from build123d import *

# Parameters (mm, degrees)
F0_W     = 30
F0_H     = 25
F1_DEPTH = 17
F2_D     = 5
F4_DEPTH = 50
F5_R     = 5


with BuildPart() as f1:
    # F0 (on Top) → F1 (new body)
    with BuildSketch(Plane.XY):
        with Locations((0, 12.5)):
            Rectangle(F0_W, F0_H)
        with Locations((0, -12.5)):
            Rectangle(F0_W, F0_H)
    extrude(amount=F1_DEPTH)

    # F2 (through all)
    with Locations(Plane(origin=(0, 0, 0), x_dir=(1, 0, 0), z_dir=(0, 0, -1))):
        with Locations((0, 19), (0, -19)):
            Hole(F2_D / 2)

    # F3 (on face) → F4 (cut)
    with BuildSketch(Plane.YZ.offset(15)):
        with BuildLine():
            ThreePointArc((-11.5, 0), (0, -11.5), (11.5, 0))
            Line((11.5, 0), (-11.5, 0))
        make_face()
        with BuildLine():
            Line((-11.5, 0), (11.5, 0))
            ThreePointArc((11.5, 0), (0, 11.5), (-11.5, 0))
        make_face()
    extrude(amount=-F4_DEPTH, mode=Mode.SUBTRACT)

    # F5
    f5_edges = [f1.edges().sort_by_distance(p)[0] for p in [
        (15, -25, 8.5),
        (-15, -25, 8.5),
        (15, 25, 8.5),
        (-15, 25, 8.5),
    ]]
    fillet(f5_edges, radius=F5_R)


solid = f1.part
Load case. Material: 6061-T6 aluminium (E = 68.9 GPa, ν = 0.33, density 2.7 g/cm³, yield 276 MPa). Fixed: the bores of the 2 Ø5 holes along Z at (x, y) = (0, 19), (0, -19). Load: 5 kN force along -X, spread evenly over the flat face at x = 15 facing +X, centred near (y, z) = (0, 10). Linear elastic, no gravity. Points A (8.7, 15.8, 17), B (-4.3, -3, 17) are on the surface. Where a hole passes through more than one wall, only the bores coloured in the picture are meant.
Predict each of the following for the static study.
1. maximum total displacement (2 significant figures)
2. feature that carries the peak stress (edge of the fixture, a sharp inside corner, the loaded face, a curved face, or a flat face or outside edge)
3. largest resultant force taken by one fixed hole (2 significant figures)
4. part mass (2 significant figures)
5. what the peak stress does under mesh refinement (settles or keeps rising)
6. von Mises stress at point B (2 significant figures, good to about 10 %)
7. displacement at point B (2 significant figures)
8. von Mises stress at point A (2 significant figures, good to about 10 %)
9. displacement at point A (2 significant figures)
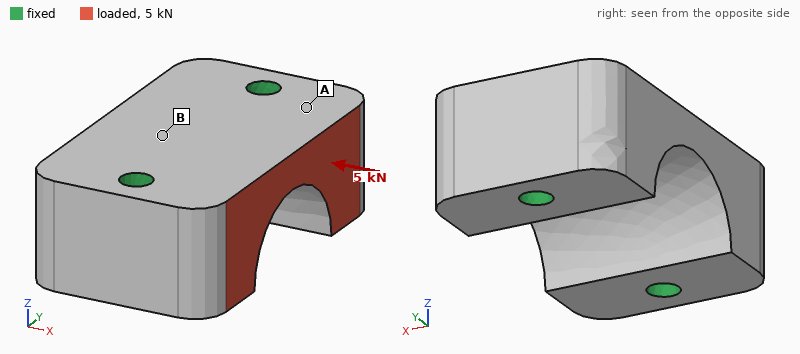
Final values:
7.1 µm
edge of the fixture
2.5 kN
49 g
keeps rising
6.3 MPa
4.2 µm
14 MPa
2.3 µm
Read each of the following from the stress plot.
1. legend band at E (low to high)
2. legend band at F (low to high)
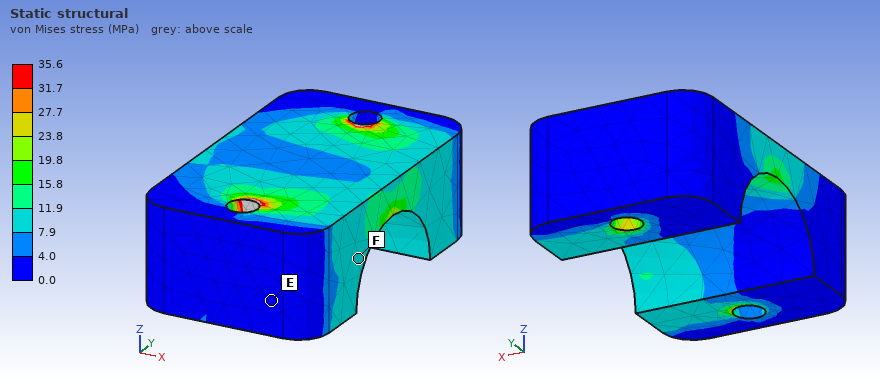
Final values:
0.0 to 4.0 MPa
7.9 to 11.9 MPa
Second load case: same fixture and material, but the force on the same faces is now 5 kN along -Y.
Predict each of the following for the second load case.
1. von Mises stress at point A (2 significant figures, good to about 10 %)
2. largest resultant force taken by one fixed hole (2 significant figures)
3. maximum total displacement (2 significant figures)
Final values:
18 MPa
2.9 kN
12 µm
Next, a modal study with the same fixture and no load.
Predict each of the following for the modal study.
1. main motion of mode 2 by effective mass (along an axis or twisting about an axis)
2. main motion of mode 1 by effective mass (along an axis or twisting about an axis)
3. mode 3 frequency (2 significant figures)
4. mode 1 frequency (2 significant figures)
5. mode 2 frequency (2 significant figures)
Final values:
along Z
along X
33 kHz
26 kHz
30 kHz
